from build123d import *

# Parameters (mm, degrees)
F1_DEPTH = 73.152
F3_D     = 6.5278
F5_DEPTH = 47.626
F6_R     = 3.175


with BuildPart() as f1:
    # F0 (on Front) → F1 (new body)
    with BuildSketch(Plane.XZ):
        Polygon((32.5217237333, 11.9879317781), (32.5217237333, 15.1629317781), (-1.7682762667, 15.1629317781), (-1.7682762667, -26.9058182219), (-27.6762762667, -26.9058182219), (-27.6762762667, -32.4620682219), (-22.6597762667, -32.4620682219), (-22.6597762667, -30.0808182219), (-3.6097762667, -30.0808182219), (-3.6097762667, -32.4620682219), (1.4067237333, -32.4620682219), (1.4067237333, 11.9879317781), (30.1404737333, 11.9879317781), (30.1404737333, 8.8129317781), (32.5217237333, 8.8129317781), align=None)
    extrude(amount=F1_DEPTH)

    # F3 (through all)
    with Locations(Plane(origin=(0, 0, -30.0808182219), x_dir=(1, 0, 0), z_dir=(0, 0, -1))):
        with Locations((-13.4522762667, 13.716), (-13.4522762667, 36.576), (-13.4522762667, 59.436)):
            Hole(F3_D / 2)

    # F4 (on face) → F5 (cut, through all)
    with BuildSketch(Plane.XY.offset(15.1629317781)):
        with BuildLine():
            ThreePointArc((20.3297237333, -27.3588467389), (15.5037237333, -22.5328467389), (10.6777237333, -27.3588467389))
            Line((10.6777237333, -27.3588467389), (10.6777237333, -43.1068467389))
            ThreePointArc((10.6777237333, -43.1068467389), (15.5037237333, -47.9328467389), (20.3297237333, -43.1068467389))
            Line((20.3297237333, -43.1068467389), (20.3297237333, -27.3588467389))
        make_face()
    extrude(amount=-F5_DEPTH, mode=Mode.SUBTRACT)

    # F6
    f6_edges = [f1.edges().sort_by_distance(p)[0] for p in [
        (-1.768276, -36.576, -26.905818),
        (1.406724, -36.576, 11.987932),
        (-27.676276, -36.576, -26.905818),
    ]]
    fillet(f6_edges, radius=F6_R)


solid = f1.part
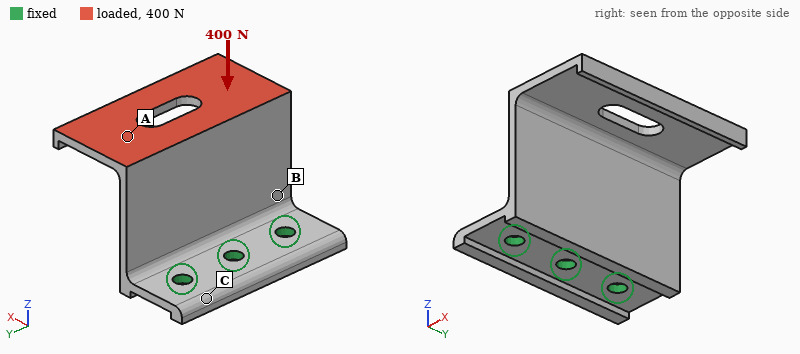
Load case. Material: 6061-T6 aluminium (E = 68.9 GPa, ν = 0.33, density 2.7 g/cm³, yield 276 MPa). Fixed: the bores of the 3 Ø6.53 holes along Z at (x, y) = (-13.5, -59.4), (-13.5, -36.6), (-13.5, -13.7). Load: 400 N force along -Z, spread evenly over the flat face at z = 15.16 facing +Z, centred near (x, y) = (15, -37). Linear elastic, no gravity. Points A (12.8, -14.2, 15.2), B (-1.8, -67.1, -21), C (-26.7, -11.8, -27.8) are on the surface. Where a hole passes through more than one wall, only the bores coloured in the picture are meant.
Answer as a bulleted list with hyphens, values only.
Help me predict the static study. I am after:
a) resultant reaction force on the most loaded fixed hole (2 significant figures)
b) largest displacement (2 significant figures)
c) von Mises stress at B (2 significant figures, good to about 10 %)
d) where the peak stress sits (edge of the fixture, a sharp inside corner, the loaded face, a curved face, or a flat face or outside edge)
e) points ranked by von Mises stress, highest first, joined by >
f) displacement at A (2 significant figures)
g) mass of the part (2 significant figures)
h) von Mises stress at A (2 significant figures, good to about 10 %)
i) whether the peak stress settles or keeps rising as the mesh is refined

- 140 N
- 1.1 mm
- 43 MPa
- edge of the fixture
- B > A > C
- 0.72 mm
- 68 g
- 26 MPa
- keeps rising
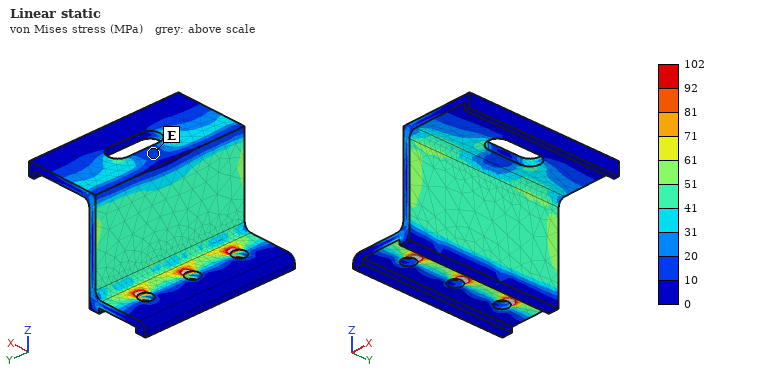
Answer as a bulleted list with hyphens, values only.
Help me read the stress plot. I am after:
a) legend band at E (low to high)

- 10 to 20 MPa
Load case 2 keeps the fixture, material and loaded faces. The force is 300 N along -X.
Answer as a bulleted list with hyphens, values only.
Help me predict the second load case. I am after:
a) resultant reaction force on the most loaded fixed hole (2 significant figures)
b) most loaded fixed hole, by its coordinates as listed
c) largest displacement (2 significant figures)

- 130 N
- (-13.5, -36.6)
- 1.3 mm
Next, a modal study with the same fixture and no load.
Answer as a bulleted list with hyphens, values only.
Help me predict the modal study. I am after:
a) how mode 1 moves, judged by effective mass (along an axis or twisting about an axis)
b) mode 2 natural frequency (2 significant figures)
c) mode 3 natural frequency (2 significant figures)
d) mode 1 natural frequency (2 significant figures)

- along X
- 1100 Hz
- 1700 Hz
- 500 Hz
